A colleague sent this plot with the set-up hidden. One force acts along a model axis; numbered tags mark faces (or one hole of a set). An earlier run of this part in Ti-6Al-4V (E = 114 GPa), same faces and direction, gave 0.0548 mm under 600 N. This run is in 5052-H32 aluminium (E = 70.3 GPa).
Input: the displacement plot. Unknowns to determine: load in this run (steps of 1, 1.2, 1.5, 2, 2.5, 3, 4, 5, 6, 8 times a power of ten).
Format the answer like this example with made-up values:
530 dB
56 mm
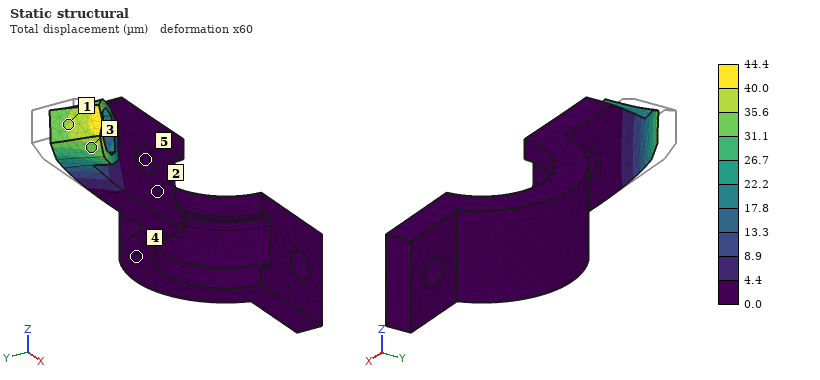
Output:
300 N
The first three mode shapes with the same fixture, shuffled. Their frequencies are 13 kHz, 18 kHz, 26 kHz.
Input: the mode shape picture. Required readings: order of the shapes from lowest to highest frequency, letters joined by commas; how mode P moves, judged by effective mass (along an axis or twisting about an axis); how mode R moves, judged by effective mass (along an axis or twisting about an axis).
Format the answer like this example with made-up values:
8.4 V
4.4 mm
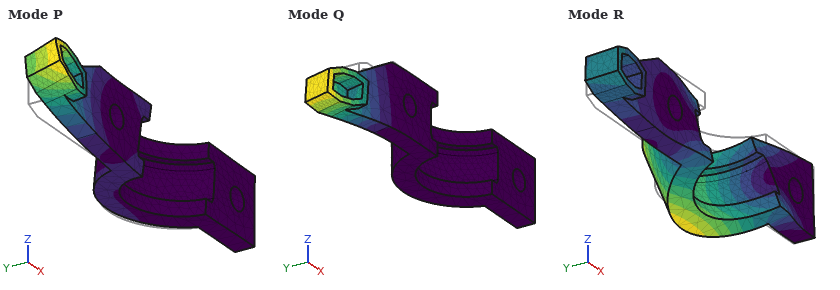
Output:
Q, R, P
along Z
along Z
